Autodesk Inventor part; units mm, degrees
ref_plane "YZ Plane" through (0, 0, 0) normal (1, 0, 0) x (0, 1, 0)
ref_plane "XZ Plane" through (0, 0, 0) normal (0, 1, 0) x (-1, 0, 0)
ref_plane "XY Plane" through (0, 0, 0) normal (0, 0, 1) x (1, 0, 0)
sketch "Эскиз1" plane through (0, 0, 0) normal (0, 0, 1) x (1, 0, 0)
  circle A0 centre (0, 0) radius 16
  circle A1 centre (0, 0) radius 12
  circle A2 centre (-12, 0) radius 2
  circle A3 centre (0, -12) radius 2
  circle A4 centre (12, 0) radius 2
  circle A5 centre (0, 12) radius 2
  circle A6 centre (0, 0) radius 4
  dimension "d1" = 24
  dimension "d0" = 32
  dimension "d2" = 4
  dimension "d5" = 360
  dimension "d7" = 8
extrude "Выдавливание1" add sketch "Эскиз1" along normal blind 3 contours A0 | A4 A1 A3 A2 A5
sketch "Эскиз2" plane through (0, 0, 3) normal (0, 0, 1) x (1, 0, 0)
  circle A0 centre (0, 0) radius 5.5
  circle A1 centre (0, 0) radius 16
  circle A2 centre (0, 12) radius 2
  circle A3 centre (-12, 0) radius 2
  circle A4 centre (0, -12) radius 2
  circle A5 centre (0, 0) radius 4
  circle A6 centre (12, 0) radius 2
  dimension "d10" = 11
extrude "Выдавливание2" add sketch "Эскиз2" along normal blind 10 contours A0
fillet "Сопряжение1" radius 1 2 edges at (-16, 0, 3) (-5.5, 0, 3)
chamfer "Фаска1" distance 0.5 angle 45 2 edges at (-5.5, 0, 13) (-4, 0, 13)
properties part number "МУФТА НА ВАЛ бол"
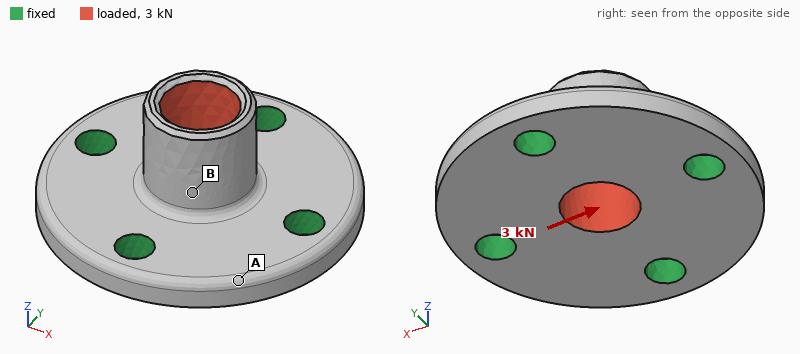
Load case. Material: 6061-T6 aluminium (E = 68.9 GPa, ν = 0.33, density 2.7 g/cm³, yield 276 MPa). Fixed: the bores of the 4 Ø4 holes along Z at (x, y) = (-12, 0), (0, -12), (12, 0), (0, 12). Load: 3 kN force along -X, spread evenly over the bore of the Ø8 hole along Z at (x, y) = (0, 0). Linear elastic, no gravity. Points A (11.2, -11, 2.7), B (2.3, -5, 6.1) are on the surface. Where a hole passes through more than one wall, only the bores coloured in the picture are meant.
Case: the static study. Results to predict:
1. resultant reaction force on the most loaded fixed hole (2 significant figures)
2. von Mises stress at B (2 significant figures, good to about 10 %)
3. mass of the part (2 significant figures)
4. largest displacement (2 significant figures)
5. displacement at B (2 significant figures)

1.2 kN
72 MPa
6.9 g
56 µm
22 µm
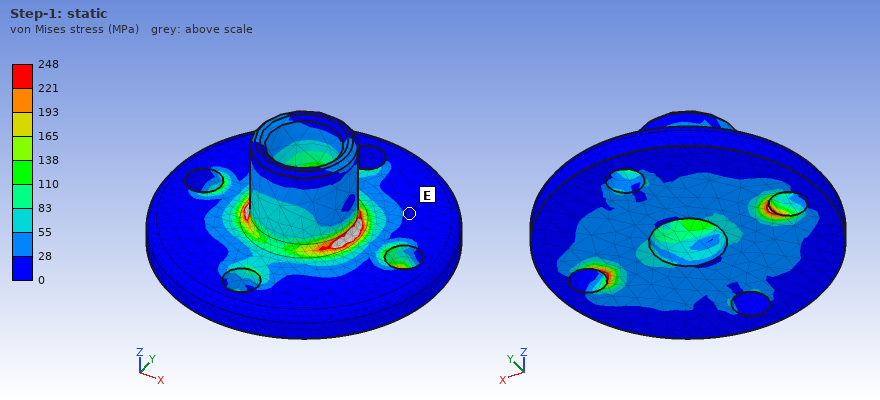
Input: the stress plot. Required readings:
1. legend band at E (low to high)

0 to 28 MPa
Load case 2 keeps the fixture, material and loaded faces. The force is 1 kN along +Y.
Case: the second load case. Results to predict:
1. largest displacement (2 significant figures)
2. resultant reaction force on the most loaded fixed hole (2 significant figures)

19 µm
420 N
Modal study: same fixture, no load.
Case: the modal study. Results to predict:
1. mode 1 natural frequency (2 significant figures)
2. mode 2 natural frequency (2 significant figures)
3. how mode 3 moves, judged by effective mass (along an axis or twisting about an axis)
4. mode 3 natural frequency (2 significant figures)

32 kHz
32 kHz
along Z
40 kHz
